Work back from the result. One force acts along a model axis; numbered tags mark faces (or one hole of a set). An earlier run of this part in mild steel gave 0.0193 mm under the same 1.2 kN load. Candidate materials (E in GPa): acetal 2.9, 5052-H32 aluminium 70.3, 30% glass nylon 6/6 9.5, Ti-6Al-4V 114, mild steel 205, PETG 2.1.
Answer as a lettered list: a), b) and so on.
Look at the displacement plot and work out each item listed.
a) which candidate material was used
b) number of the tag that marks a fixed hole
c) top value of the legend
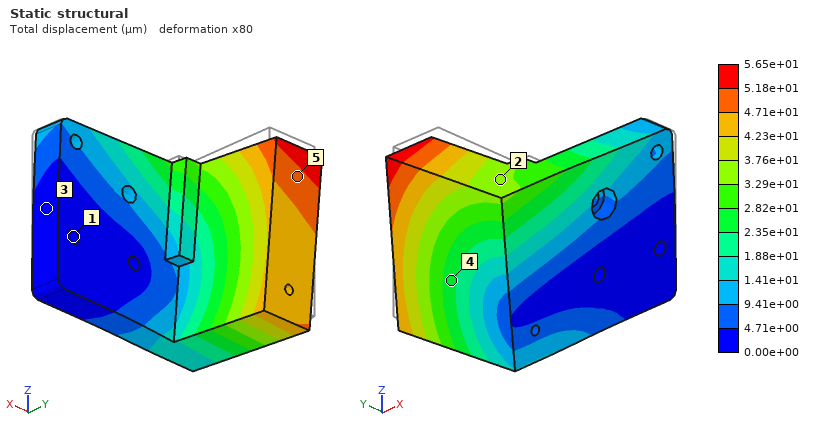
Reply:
a) 5052-H32 aluminium
b) 1
c) 5.65e+01 µm
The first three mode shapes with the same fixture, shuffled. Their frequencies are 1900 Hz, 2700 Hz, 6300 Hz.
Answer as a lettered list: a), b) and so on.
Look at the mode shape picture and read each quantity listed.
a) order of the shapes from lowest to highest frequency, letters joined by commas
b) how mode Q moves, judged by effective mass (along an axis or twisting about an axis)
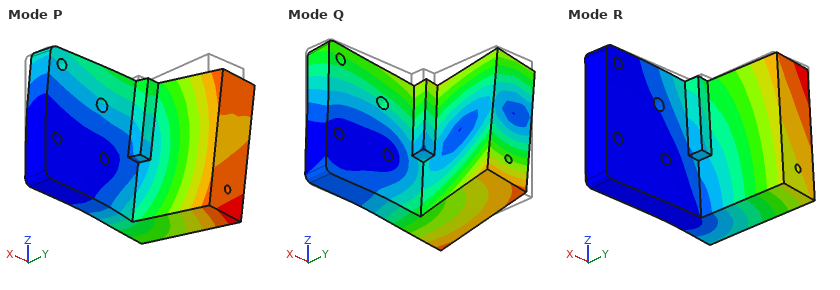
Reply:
a) R, P, Q
b) along Z
